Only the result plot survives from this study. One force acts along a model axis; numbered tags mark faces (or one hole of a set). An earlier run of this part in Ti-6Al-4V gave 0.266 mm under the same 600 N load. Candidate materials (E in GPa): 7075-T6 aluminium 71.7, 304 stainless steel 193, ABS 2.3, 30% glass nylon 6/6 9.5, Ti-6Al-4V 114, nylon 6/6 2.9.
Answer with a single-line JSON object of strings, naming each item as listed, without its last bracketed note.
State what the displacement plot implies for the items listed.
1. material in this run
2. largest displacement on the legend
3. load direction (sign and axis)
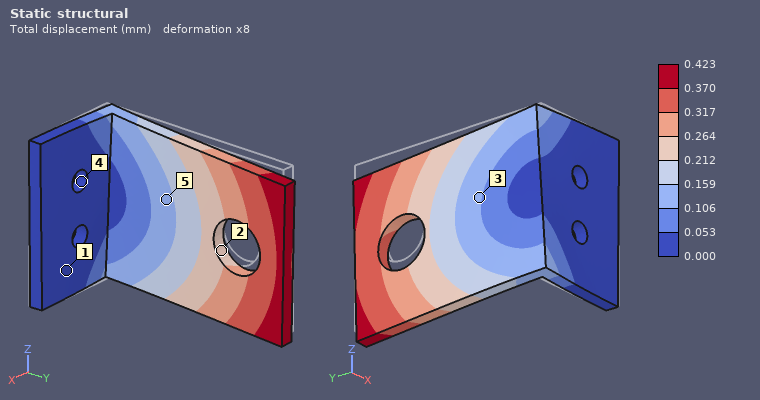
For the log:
{"material in this run": "7075-T6 aluminium", "largest displacement on the legend": "0.423 mm", "load direction": "-Z"}
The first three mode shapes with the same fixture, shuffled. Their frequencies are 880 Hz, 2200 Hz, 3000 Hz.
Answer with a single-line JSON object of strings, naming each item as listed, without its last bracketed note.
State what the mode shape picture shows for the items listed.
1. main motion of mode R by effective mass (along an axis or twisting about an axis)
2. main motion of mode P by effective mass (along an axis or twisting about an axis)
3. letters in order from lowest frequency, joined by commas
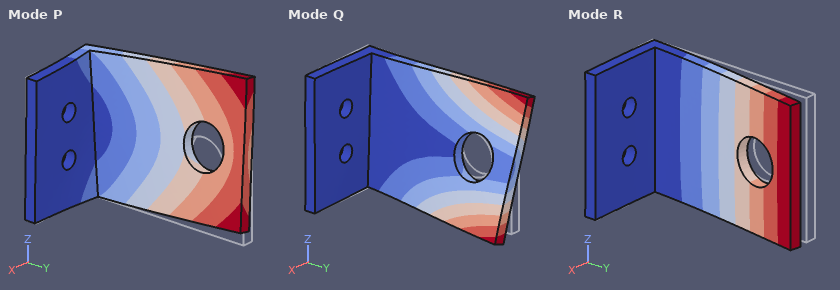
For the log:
{"main motion of mode R by effective mass": "along X", "main motion of mode P by effective mass": "along Z", "letters in order from lowest frequency, joined by commas": "R, P, Q"}
